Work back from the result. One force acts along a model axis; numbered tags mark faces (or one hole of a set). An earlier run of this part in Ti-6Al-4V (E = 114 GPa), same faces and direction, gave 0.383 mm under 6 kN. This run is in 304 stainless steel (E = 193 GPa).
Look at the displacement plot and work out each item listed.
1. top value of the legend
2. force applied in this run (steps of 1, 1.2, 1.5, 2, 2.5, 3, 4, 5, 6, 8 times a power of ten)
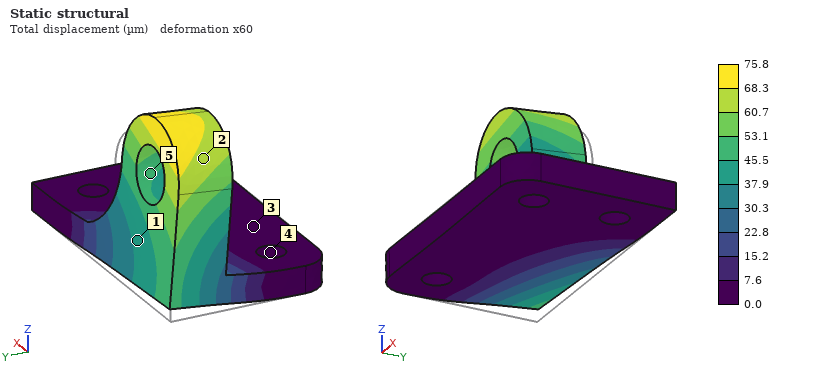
75.8 µm
2 kN
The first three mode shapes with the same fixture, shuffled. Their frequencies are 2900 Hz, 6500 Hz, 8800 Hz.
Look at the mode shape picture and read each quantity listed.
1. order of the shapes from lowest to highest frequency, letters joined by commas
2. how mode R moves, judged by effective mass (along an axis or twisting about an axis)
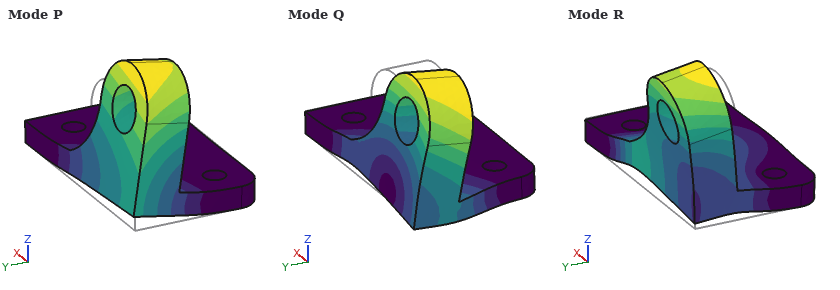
P, Q, R
along Z
